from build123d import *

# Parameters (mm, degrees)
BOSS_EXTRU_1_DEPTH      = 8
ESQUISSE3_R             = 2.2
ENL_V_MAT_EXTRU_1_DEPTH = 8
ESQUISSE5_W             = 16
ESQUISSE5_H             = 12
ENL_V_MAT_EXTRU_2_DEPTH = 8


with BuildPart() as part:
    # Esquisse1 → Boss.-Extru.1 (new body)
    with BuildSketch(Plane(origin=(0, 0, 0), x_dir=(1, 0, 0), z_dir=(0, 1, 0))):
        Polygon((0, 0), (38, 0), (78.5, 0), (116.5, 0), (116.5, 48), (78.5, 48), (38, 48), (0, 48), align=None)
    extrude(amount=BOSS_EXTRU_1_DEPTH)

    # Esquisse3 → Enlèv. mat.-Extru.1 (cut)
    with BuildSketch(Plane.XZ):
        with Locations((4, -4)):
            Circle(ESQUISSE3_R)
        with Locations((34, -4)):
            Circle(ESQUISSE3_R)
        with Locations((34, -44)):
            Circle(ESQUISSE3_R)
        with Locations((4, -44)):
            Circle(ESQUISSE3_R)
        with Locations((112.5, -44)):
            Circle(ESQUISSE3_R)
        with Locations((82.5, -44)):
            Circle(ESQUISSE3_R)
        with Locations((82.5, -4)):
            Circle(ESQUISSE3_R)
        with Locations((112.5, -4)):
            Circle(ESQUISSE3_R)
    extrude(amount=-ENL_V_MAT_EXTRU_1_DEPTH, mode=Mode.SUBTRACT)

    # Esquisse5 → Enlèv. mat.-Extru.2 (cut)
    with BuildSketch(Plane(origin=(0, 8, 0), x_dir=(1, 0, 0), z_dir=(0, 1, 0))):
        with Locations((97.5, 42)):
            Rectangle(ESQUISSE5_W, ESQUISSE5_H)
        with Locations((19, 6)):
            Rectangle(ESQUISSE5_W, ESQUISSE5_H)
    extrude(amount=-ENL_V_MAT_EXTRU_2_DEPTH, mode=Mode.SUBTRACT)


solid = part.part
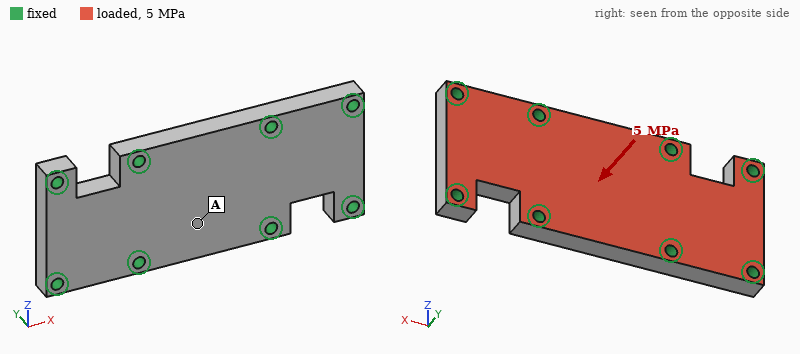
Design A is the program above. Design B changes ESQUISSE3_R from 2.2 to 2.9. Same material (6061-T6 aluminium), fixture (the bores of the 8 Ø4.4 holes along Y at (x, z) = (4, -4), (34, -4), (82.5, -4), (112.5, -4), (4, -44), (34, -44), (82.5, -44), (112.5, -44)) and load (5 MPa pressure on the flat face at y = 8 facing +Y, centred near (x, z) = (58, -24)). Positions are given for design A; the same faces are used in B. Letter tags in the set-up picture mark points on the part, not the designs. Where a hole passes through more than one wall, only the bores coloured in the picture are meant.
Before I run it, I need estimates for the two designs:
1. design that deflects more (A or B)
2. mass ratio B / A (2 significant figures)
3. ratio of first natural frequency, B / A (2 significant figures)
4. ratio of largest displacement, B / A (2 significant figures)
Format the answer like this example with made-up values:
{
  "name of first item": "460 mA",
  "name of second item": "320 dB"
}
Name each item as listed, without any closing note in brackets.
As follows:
{
  "design that deflects more": "A",
  "mass ratio B / A": "0.98",
  "ratio of first natural frequency, B / A": "1.1",
  "ratio of largest displacement, B / A": "0.87"
}
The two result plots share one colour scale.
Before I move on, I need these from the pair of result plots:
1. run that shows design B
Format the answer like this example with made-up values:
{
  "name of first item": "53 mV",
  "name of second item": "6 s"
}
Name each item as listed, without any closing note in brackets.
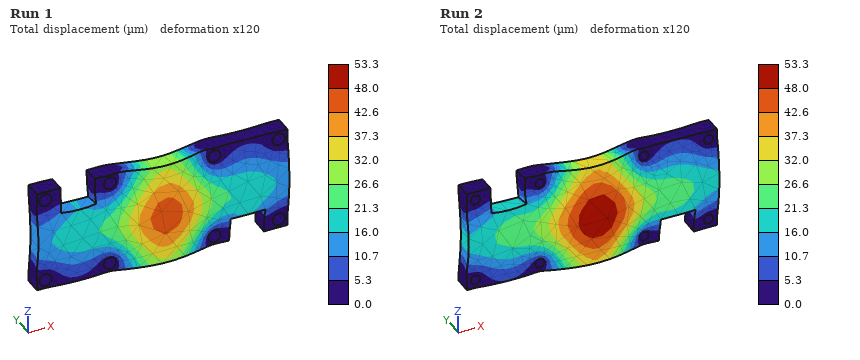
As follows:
{
  "run that shows design B": "Run 1"
}
